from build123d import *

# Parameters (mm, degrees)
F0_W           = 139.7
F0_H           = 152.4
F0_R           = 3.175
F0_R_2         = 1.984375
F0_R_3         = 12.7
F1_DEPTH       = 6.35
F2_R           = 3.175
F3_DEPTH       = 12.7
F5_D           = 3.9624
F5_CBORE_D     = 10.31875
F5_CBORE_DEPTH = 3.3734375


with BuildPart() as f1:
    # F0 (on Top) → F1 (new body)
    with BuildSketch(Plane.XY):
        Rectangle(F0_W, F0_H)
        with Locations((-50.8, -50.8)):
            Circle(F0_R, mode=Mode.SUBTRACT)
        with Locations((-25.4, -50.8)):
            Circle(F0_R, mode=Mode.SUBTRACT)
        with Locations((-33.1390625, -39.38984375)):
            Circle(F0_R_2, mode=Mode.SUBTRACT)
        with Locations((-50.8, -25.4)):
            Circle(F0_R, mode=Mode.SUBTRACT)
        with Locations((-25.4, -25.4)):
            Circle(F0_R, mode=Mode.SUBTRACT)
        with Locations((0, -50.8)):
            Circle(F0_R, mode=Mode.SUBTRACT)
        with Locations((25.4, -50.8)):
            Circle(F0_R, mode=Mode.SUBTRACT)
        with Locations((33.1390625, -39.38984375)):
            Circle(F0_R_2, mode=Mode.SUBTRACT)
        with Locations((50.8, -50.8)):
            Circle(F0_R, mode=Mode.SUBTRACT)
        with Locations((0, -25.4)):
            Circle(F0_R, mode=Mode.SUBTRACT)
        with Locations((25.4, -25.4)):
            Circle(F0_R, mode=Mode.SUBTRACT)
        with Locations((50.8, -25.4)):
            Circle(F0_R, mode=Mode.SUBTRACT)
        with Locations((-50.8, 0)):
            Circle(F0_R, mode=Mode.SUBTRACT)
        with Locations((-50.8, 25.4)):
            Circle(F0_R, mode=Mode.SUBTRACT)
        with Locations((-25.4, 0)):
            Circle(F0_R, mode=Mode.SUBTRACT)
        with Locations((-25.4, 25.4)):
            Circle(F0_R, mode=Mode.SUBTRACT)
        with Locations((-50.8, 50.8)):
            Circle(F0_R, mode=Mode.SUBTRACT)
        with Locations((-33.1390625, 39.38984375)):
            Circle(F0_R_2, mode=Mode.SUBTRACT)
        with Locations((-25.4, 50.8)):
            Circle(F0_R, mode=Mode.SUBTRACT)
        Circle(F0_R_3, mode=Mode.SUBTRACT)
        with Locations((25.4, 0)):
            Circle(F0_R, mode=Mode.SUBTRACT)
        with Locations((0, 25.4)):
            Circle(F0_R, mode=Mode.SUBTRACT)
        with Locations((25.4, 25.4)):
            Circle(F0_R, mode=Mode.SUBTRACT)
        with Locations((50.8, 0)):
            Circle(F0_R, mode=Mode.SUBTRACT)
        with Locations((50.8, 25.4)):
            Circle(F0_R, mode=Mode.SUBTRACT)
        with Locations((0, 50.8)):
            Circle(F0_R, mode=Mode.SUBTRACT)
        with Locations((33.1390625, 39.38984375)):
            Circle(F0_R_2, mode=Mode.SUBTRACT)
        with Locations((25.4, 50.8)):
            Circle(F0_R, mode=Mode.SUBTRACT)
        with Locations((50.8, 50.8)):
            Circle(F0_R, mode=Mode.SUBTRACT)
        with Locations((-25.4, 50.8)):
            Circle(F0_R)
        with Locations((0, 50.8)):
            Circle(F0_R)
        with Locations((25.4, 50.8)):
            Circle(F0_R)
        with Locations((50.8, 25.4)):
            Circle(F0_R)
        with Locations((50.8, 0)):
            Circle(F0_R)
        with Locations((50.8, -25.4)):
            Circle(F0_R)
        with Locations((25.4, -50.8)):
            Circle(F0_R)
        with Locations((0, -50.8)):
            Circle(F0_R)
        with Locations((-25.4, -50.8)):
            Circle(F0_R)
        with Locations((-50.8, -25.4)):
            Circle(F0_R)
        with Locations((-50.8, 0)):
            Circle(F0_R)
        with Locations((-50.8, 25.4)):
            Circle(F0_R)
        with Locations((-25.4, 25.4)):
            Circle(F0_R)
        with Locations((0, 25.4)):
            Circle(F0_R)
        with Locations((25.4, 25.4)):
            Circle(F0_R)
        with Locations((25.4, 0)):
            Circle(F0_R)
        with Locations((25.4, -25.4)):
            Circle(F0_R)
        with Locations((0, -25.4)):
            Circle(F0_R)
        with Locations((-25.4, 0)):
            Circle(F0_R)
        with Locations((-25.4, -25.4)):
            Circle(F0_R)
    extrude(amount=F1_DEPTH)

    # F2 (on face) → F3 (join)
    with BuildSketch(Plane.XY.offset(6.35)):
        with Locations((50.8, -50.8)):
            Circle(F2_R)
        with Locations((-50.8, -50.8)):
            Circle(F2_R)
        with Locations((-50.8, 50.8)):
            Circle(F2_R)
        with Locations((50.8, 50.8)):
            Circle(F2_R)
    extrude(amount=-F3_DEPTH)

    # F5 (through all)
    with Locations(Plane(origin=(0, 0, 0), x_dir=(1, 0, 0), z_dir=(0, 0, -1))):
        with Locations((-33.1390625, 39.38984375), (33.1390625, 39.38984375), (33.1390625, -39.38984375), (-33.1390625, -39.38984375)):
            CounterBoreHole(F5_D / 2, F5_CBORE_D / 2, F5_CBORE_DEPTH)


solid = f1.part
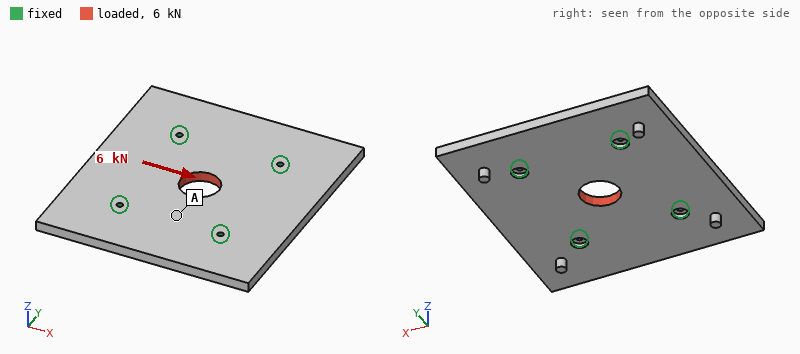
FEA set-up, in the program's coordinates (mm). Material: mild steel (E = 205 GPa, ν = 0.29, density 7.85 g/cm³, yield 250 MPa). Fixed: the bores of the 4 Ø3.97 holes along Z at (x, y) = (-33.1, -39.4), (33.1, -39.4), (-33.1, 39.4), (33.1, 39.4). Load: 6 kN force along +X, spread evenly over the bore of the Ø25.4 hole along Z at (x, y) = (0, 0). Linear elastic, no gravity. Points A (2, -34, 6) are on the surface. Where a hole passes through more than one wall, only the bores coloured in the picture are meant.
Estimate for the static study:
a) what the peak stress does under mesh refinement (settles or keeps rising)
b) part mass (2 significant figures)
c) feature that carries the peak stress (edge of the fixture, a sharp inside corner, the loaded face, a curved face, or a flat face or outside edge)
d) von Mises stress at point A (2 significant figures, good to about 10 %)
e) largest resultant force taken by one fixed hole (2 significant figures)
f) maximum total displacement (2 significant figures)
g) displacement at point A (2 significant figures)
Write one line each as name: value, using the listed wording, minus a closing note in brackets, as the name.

what the peak stress does under mesh refinement: keeps rising
part mass: 1.0 kg
feature that carries the peak stress: edge of the fixture
von Mises stress at point A: 5.1 MPa
largest resultant force taken by one fixed hole: 1.5 kN
maximum total displacement: 3.8 µm
displacement at point A: 1.6 µm
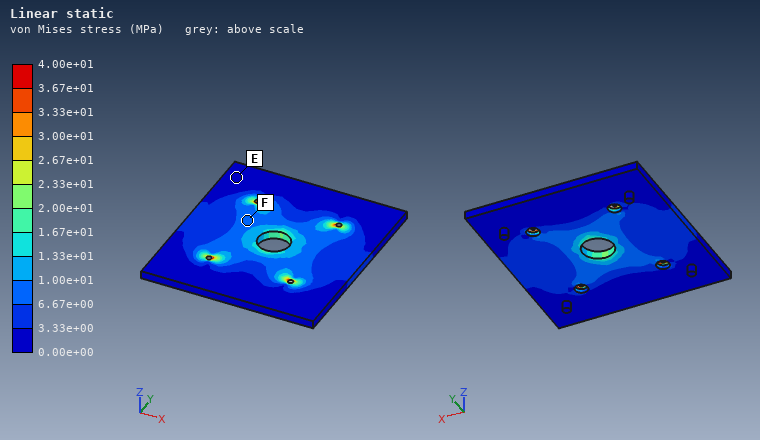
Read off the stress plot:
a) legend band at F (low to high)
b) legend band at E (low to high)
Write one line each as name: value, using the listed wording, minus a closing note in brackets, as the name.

legend band at F: 6.67e+00 to 1.00e+01 MPa
legend band at E: 0.00e+00 to 3.33e+00 MPa
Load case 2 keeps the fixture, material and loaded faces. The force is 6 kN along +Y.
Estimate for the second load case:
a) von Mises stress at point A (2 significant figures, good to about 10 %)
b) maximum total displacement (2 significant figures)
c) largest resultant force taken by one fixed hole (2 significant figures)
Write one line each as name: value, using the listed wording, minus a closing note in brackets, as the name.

von Mises stress at point A: 7.7 MPa
maximum total displacement: 4.1 µm
largest resultant force taken by one fixed hole: 1.5 kN
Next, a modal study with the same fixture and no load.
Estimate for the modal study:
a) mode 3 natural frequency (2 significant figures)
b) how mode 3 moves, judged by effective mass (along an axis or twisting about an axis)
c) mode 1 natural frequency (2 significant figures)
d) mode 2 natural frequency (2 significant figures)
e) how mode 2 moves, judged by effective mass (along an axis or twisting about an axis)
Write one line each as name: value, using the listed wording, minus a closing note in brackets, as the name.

mode 3 natural frequency: 2300 Hz
how mode 3 moves, judged by effective mass: twisting about Y
mode 1 natural frequency: 1900 Hz
mode 2 natural frequency: 2000 Hz
how mode 2 moves, judged by effective mass: along Z
